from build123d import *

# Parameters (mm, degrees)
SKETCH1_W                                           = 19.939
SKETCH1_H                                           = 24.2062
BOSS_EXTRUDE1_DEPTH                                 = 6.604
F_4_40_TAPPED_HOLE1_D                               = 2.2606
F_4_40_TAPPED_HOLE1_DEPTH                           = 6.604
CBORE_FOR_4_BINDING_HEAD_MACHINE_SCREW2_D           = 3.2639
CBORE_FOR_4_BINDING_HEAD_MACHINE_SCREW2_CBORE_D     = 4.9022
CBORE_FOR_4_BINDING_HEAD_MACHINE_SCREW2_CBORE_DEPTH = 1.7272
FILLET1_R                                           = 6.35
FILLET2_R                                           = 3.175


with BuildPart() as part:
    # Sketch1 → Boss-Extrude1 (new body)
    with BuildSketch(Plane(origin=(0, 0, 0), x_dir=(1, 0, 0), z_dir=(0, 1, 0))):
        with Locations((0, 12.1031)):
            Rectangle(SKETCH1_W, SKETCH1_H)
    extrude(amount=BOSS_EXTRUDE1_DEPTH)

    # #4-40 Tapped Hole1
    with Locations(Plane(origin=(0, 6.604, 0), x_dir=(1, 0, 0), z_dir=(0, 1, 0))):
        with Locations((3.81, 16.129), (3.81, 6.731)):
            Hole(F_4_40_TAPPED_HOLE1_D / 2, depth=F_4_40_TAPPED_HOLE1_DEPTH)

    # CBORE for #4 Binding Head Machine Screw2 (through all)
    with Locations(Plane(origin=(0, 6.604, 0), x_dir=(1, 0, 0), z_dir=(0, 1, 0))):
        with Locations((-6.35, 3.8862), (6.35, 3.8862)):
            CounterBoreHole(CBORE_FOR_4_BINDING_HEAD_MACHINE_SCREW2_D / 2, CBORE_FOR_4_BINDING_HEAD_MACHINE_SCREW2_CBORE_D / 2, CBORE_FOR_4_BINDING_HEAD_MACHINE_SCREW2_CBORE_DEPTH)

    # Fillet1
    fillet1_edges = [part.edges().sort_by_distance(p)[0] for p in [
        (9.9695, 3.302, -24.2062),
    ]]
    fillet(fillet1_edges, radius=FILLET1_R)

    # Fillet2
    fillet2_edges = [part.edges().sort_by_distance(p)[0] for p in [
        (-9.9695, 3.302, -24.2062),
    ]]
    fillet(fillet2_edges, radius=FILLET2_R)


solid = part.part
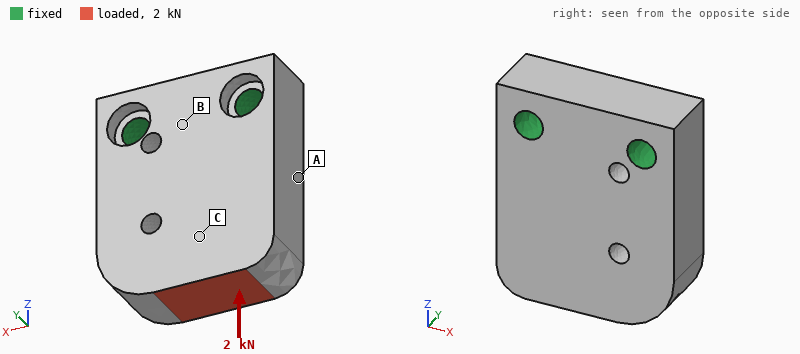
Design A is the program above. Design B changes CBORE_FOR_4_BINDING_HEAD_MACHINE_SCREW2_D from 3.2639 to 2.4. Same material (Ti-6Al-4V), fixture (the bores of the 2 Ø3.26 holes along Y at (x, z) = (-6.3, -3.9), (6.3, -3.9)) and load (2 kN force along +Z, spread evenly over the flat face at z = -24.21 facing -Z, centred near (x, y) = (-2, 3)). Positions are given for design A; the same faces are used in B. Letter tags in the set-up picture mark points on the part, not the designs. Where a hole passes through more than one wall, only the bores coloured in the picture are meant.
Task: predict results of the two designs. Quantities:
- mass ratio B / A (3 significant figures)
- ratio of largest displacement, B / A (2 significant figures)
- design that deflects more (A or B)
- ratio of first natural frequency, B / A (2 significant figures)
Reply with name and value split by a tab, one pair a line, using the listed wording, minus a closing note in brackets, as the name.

mass ratio B / A	1.01
ratio of largest displacement, B / A	1.2
design that deflects more	B
ratio of first natural frequency, B / A	0.91
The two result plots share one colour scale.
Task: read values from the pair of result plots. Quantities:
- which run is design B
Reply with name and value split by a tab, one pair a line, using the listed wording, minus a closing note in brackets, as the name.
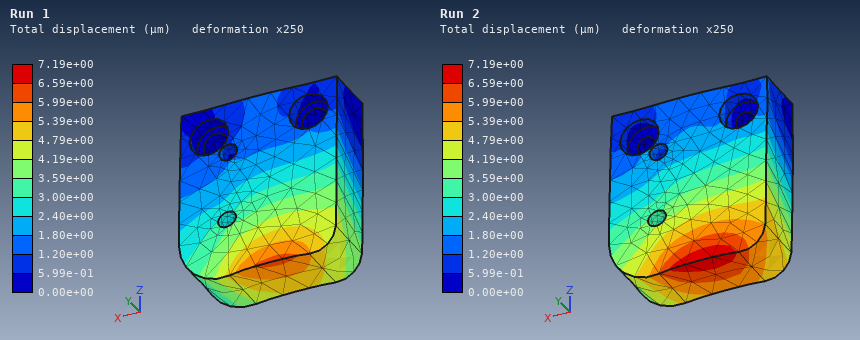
which run is design B	Run 2
